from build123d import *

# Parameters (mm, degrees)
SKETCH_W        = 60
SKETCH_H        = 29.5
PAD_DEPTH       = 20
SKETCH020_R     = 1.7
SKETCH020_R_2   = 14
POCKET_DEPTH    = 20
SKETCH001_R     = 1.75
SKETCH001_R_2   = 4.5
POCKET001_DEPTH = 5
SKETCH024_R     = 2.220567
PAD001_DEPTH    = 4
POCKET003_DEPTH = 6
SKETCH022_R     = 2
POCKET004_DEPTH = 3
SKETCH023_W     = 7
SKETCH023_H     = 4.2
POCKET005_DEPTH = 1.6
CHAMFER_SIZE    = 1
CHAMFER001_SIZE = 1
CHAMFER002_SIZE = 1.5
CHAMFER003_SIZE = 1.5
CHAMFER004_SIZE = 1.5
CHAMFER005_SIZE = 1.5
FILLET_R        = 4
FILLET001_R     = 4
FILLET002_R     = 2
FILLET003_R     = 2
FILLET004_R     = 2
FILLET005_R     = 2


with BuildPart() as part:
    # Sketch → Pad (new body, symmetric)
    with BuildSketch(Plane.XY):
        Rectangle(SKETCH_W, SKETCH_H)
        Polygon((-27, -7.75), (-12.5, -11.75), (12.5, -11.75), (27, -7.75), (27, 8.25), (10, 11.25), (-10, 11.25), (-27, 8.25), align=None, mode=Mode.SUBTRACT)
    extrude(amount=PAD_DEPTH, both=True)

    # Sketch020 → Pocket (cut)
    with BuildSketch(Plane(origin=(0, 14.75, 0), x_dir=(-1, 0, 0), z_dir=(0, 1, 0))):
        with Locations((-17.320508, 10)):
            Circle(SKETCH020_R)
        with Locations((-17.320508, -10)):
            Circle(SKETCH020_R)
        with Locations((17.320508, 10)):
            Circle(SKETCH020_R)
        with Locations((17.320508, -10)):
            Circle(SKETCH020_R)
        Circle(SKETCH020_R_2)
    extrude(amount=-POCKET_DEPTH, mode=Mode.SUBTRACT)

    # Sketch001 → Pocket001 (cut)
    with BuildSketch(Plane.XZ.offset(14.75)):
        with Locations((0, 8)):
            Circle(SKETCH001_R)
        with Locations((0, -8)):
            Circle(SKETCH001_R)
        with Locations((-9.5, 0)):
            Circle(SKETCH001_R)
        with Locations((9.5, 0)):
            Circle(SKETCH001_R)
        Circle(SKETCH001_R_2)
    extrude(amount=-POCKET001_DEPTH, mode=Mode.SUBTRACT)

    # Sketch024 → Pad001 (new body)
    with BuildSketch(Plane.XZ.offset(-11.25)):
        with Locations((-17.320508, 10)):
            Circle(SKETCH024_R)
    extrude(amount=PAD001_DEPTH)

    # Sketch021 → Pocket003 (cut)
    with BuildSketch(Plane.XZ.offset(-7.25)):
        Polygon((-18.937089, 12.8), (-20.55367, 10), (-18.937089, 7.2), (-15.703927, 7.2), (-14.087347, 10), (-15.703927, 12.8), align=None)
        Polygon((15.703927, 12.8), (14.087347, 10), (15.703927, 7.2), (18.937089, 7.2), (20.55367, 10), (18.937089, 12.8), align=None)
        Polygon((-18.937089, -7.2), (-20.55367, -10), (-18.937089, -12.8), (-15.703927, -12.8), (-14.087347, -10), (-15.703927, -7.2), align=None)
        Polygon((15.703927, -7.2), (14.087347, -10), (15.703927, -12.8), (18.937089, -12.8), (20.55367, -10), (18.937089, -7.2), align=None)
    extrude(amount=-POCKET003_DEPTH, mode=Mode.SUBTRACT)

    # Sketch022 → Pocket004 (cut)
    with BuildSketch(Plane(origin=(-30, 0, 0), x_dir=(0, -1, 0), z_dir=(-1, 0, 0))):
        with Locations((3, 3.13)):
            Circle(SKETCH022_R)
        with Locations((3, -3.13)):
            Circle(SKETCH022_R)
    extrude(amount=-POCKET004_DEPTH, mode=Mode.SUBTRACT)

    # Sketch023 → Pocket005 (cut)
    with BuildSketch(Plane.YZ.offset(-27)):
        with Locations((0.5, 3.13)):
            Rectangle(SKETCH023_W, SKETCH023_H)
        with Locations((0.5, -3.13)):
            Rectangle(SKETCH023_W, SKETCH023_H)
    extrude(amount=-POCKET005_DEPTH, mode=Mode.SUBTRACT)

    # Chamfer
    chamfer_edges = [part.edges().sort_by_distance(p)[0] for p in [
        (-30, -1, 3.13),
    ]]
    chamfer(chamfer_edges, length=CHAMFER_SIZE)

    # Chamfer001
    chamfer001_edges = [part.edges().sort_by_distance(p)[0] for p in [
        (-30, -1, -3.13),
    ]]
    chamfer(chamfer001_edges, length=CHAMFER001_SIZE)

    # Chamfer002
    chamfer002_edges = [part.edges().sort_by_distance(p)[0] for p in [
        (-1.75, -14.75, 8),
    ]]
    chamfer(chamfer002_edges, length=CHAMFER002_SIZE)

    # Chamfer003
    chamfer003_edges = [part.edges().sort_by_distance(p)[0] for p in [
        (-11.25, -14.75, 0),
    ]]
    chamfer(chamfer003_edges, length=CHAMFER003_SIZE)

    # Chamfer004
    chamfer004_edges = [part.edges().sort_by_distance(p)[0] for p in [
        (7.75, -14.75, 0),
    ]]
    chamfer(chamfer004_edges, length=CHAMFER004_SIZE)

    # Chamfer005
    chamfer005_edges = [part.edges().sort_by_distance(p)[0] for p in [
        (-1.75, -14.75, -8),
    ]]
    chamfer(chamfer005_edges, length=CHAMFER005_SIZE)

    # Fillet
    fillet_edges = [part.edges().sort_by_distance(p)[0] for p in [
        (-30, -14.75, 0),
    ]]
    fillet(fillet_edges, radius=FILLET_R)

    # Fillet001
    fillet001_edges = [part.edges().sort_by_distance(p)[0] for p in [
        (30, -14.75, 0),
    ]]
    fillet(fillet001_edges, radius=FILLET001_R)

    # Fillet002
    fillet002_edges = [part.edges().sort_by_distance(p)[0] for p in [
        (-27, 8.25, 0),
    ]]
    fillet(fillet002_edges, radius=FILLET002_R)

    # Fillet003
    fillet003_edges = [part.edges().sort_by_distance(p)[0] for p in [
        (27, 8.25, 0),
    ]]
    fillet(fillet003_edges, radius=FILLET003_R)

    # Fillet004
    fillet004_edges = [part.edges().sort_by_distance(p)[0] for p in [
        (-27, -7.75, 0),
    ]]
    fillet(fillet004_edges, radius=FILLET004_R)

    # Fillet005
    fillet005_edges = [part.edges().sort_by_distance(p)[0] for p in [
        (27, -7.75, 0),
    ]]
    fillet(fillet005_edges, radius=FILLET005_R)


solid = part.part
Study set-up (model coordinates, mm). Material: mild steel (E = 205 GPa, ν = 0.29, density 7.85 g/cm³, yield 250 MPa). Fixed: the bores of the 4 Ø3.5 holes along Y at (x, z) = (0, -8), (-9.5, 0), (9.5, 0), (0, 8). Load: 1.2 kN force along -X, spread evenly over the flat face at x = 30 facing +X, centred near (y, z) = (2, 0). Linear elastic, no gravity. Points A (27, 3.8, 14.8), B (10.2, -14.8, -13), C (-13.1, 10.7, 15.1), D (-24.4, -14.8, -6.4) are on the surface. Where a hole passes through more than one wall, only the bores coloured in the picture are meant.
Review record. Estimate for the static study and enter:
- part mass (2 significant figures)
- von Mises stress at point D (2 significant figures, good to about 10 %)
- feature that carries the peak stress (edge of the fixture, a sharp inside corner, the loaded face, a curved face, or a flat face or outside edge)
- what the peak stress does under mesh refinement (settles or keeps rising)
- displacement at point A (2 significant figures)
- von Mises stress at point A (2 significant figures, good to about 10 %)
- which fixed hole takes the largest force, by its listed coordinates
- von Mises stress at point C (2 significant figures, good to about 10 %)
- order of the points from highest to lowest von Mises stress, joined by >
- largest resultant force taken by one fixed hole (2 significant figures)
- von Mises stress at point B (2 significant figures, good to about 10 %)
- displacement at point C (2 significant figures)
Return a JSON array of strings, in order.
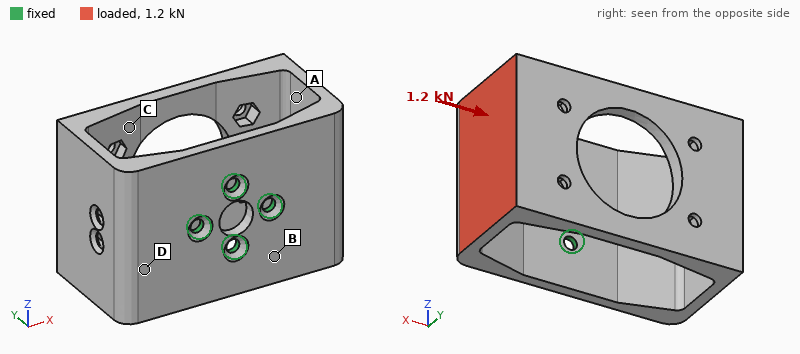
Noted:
["170 g", "17 MPa", "edge of the fixture", "keeps rising", "0.10 mm", "58 MPa", "(9.5, 0)", "44 MPa", "B > A > C > D", "1.1 kN", "90 MPa", "0.094 mm"]
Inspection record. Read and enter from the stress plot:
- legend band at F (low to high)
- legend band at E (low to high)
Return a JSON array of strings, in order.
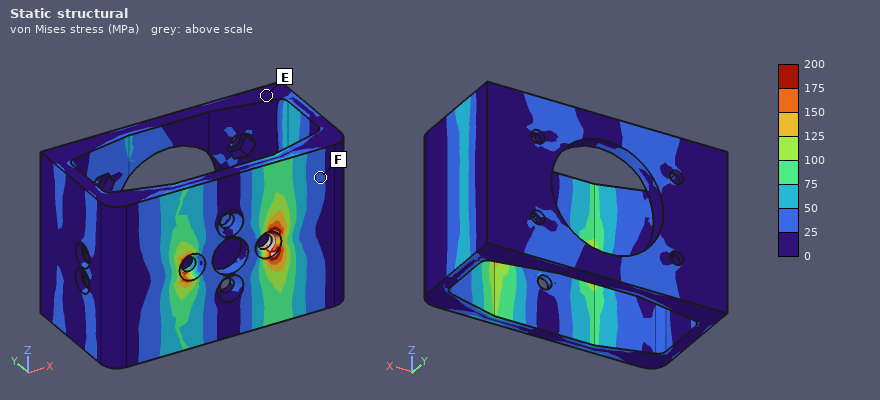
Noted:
["25 to 50 MPa", "0 to 25 MPa"]
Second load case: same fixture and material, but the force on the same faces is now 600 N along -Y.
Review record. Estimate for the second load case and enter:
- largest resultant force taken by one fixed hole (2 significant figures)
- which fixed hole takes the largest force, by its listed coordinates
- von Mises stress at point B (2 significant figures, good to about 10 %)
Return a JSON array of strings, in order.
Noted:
["1.1 kN", "(9.5, 0)", "73 MPa"]
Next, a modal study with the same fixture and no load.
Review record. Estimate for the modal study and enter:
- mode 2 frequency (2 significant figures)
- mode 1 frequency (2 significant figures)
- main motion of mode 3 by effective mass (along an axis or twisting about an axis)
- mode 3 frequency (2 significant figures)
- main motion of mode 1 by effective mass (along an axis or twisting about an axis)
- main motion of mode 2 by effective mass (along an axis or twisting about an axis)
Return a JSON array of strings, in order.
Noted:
["1500 Hz", "1200 Hz", "along Y", "2100 Hz", "along X", "along Z"]
